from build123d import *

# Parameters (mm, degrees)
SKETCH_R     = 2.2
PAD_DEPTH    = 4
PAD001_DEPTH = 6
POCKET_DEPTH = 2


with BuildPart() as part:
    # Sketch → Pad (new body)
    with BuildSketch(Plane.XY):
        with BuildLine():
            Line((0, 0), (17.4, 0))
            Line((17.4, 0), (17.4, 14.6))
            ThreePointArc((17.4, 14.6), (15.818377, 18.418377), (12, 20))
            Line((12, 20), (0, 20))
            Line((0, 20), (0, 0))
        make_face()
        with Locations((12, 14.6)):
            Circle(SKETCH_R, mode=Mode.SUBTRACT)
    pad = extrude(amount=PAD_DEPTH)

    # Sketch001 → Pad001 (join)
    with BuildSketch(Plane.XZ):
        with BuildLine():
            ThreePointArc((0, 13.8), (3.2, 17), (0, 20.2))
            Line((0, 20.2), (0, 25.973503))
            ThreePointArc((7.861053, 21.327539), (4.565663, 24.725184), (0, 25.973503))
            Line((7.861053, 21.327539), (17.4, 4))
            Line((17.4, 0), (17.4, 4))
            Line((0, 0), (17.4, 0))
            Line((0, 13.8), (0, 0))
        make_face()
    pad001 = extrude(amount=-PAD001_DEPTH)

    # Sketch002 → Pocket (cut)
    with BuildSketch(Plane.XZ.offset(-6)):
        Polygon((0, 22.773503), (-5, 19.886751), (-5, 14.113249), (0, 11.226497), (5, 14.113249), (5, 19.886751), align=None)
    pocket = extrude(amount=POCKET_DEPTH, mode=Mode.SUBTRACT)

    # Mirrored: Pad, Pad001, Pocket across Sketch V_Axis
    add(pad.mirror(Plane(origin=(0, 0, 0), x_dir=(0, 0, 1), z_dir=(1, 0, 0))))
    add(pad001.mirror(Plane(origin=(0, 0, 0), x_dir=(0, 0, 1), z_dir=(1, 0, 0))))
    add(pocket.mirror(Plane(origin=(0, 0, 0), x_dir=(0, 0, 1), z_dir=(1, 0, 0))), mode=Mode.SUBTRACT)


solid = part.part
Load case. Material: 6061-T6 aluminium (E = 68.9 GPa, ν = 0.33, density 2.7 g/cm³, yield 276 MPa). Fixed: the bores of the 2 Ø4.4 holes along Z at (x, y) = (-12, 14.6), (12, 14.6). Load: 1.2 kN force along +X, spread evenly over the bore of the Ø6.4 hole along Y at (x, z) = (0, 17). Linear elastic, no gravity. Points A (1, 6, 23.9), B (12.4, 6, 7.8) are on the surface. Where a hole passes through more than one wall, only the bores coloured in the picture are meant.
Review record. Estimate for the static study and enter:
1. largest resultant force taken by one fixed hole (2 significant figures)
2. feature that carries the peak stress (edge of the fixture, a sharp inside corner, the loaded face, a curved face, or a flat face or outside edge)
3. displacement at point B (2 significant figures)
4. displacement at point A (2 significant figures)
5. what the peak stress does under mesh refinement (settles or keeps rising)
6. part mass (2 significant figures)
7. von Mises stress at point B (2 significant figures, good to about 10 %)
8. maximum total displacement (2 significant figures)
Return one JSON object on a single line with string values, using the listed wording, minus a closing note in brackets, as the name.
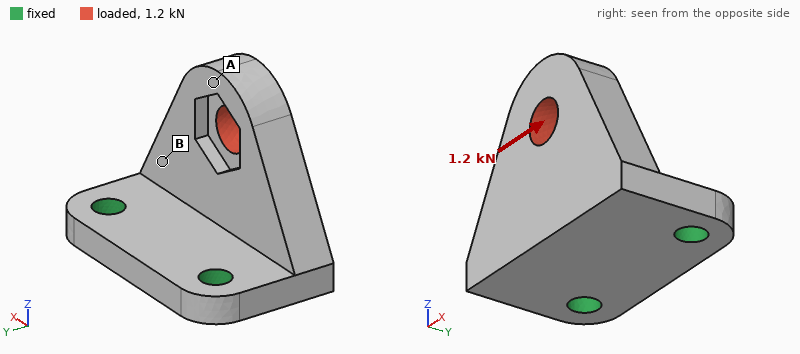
{"largest resultant force taken by one fixed hole": "1.1 kN", "feature that carries the peak stress": "edge of the fixture", "displacement at point B": "27 µm", "displacement at point A": "54 µm", "what the peak stress does under mesh refinement": "keeps rising", "part mass": "14 g", "von Mises stress at point B": "43 MPa", "maximum total displacement": "57 µm"}
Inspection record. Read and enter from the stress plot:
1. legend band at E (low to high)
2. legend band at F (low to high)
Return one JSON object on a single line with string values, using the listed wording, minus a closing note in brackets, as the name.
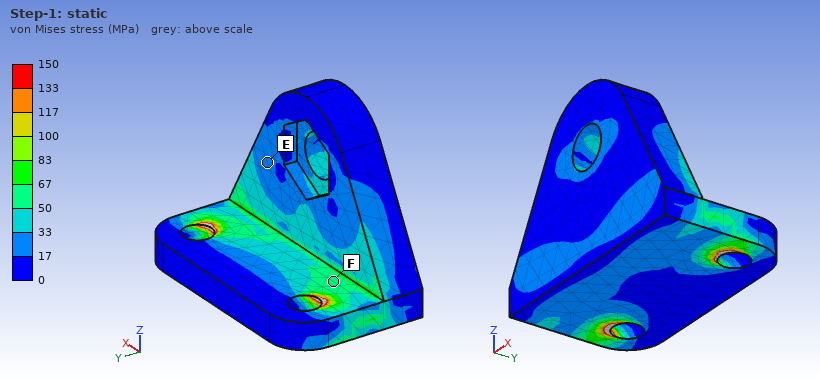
{"legend band at E": "17 to 33 MPa", "legend band at F": "50 to 67 MPa"}
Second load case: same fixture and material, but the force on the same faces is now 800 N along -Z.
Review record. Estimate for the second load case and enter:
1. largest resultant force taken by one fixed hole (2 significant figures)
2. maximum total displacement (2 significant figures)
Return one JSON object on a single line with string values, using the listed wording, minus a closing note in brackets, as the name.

{"largest resultant force taken by one fixed hole": "400 N", "maximum total displacement": "0.13 mm"}
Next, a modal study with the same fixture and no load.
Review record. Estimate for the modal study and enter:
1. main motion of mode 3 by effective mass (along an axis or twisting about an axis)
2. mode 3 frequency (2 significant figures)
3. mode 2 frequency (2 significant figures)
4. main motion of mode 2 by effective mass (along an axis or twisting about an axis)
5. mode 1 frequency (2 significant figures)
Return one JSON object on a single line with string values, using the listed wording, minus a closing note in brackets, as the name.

{"main motion of mode 3 by effective mass": "along Z", "mode 3 frequency": "15 kHz", "mode 2 frequency": "11 kHz", "main motion of mode 2 by effective mass": "along X", "mode 1 frequency": "4500 Hz"}
